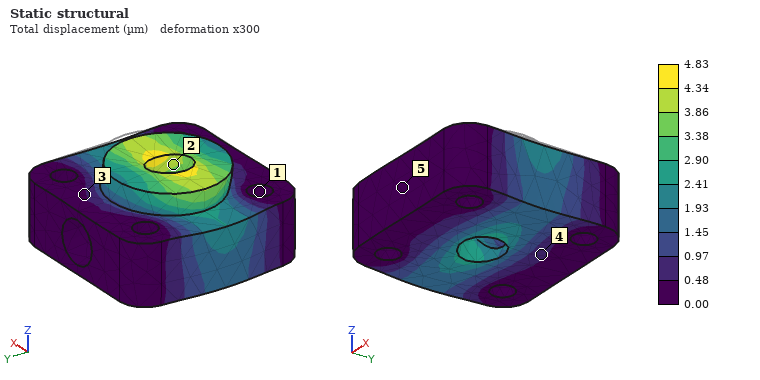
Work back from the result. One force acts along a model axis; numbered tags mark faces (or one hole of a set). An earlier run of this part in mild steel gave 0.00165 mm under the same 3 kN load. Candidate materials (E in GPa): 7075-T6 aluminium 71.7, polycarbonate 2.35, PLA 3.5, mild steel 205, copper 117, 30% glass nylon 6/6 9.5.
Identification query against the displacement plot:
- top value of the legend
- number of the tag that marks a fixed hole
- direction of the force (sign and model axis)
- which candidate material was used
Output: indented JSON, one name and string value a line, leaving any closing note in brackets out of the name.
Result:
{
  "top value of the legend": "4.83 µm",
  "number of the tag that marks a fixed hole": "1",
  "direction of the force": "-X",
  "which candidate material was used": "7075-T6 aluminium"
}
